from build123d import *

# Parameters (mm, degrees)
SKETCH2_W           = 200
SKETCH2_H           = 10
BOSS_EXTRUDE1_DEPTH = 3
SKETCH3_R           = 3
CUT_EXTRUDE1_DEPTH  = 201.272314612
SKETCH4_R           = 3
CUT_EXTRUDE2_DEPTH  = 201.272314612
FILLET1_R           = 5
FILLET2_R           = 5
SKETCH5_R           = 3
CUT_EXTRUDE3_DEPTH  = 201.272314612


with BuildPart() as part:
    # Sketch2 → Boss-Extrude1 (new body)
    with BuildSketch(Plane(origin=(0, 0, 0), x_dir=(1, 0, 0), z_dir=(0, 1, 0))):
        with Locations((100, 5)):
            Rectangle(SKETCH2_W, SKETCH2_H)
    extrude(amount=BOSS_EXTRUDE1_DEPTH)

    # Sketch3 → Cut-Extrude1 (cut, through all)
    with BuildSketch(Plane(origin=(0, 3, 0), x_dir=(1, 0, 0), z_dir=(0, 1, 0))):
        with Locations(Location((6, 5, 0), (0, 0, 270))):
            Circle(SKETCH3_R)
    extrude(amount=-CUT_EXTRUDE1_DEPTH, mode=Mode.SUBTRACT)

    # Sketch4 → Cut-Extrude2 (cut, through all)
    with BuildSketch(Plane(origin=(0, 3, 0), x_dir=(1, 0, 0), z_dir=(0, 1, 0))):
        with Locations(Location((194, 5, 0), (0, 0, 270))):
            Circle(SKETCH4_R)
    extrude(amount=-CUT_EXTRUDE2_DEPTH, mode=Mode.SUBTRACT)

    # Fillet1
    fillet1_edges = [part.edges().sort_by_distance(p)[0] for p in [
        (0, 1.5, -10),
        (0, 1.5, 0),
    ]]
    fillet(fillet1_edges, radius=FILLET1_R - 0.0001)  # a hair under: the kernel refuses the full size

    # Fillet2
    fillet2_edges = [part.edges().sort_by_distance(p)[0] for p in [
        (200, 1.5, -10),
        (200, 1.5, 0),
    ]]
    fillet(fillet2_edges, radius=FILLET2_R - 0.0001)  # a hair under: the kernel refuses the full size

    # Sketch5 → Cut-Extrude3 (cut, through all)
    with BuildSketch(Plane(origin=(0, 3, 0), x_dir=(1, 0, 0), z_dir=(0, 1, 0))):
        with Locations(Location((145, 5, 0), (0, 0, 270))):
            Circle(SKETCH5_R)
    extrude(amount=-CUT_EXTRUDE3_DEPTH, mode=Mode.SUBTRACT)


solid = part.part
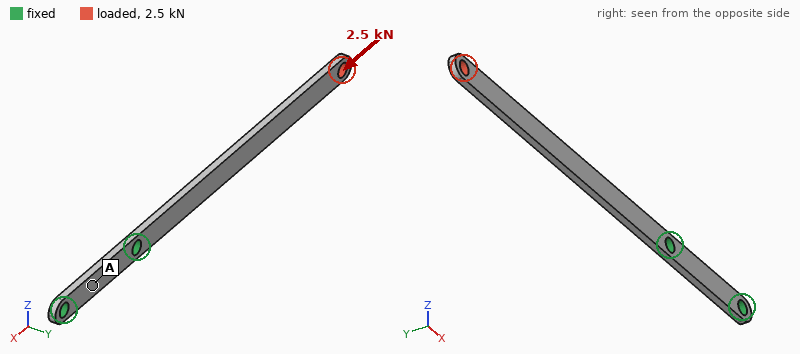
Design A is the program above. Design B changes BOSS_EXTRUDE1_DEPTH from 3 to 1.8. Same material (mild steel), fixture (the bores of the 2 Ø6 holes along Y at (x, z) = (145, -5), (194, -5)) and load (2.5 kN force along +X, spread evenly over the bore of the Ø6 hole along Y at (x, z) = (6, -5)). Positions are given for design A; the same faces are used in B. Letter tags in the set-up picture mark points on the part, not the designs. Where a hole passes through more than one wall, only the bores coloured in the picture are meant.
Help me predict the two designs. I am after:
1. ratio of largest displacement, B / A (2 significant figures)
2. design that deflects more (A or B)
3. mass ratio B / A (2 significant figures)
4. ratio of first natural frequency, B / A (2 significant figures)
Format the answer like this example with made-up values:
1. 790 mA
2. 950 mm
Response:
1. 1.7
2. B
3. 0.60
4. 0.60
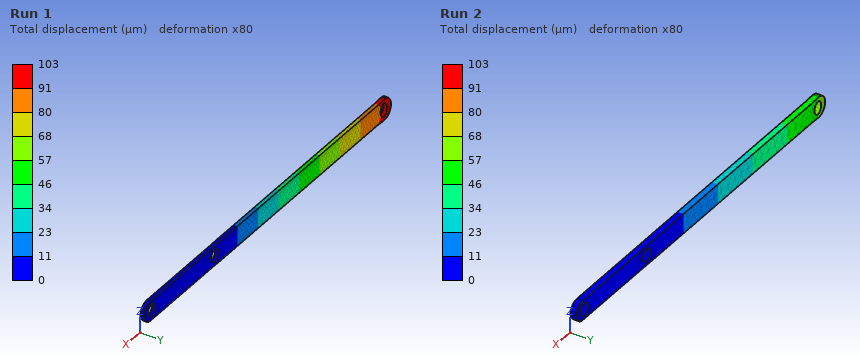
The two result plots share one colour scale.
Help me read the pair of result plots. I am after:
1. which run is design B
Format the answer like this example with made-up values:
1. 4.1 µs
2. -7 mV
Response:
1. Run 1
